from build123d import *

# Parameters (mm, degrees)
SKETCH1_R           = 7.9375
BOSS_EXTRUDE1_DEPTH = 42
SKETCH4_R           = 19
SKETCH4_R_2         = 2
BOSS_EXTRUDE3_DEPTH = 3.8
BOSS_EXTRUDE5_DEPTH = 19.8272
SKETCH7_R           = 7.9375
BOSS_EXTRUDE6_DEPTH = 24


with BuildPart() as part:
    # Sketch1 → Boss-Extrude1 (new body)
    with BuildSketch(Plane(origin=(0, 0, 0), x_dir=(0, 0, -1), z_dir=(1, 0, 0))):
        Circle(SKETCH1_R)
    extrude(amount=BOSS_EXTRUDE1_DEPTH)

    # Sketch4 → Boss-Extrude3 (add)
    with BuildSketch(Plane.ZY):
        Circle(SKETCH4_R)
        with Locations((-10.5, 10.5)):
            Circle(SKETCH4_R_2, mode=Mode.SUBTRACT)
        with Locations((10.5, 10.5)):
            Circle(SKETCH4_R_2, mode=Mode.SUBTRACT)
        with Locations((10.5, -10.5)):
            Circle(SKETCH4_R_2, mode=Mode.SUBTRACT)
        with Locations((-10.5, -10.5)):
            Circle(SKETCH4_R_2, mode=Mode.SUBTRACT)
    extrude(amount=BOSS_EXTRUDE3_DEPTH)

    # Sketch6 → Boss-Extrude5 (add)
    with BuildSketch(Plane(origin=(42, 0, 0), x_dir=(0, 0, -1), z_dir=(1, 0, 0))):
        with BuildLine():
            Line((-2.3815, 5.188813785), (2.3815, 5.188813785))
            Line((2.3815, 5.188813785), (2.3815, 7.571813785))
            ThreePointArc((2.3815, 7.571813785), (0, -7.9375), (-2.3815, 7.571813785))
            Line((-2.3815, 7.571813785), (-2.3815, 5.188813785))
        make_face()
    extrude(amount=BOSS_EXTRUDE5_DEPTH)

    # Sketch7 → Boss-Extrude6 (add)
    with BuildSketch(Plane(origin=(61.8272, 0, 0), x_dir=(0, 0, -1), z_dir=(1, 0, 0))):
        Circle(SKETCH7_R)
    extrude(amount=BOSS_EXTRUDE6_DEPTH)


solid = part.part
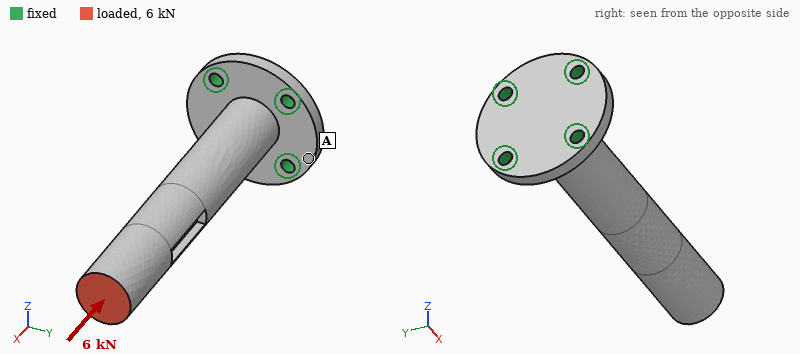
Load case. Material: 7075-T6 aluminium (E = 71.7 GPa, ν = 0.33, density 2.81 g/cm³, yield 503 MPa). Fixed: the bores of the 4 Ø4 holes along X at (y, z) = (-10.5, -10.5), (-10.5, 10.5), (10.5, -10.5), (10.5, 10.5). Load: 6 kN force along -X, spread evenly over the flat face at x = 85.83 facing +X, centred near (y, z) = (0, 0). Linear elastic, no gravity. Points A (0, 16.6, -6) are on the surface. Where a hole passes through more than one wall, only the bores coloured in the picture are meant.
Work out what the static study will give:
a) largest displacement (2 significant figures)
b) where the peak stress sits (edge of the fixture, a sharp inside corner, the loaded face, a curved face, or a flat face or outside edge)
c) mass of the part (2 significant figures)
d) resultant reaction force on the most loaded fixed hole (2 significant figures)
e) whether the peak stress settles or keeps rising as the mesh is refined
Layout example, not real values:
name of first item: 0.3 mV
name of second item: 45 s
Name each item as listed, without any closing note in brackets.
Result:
largest displacement: 65 µm
where the peak stress sits: edge of the fixture
mass of the part: 59 g
resultant reaction force on the most loaded fixed hole: 1.6 kN
whether the peak stress settles or keeps rising as the mesh is refined: keeps rising
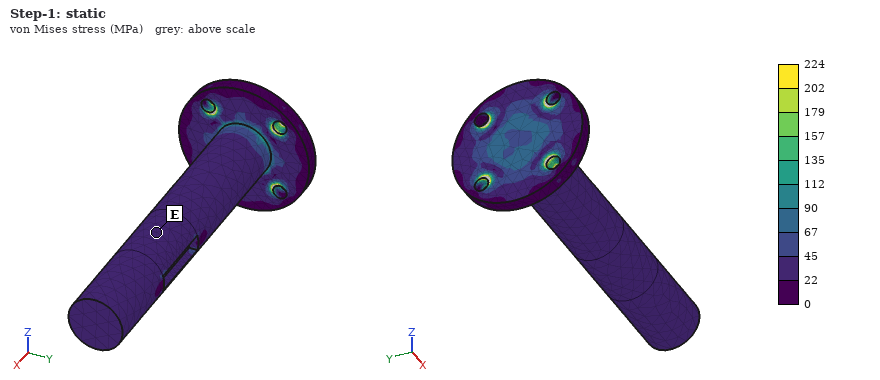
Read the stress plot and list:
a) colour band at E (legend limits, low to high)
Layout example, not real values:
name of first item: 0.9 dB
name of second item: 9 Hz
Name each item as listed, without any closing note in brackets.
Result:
colour band at E: 22 to 45 MPa
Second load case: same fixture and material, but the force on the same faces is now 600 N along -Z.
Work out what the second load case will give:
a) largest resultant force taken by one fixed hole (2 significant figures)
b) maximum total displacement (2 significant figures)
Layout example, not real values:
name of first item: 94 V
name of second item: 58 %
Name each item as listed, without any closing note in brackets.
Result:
largest resultant force taken by one fixed hole: 1.5 kN
maximum total displacement: 0.86 mm
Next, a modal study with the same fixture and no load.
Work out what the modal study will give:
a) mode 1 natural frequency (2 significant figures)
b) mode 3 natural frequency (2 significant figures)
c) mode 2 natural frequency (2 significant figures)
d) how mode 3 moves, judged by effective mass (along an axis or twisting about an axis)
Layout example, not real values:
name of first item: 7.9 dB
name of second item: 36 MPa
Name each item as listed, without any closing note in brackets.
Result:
mode 1 natural frequency: 1200 Hz
mode 3 natural frequency: 7000 Hz
mode 2 natural frequency: 1200 Hz
how mode 3 moves, judged by effective mass: along Y
